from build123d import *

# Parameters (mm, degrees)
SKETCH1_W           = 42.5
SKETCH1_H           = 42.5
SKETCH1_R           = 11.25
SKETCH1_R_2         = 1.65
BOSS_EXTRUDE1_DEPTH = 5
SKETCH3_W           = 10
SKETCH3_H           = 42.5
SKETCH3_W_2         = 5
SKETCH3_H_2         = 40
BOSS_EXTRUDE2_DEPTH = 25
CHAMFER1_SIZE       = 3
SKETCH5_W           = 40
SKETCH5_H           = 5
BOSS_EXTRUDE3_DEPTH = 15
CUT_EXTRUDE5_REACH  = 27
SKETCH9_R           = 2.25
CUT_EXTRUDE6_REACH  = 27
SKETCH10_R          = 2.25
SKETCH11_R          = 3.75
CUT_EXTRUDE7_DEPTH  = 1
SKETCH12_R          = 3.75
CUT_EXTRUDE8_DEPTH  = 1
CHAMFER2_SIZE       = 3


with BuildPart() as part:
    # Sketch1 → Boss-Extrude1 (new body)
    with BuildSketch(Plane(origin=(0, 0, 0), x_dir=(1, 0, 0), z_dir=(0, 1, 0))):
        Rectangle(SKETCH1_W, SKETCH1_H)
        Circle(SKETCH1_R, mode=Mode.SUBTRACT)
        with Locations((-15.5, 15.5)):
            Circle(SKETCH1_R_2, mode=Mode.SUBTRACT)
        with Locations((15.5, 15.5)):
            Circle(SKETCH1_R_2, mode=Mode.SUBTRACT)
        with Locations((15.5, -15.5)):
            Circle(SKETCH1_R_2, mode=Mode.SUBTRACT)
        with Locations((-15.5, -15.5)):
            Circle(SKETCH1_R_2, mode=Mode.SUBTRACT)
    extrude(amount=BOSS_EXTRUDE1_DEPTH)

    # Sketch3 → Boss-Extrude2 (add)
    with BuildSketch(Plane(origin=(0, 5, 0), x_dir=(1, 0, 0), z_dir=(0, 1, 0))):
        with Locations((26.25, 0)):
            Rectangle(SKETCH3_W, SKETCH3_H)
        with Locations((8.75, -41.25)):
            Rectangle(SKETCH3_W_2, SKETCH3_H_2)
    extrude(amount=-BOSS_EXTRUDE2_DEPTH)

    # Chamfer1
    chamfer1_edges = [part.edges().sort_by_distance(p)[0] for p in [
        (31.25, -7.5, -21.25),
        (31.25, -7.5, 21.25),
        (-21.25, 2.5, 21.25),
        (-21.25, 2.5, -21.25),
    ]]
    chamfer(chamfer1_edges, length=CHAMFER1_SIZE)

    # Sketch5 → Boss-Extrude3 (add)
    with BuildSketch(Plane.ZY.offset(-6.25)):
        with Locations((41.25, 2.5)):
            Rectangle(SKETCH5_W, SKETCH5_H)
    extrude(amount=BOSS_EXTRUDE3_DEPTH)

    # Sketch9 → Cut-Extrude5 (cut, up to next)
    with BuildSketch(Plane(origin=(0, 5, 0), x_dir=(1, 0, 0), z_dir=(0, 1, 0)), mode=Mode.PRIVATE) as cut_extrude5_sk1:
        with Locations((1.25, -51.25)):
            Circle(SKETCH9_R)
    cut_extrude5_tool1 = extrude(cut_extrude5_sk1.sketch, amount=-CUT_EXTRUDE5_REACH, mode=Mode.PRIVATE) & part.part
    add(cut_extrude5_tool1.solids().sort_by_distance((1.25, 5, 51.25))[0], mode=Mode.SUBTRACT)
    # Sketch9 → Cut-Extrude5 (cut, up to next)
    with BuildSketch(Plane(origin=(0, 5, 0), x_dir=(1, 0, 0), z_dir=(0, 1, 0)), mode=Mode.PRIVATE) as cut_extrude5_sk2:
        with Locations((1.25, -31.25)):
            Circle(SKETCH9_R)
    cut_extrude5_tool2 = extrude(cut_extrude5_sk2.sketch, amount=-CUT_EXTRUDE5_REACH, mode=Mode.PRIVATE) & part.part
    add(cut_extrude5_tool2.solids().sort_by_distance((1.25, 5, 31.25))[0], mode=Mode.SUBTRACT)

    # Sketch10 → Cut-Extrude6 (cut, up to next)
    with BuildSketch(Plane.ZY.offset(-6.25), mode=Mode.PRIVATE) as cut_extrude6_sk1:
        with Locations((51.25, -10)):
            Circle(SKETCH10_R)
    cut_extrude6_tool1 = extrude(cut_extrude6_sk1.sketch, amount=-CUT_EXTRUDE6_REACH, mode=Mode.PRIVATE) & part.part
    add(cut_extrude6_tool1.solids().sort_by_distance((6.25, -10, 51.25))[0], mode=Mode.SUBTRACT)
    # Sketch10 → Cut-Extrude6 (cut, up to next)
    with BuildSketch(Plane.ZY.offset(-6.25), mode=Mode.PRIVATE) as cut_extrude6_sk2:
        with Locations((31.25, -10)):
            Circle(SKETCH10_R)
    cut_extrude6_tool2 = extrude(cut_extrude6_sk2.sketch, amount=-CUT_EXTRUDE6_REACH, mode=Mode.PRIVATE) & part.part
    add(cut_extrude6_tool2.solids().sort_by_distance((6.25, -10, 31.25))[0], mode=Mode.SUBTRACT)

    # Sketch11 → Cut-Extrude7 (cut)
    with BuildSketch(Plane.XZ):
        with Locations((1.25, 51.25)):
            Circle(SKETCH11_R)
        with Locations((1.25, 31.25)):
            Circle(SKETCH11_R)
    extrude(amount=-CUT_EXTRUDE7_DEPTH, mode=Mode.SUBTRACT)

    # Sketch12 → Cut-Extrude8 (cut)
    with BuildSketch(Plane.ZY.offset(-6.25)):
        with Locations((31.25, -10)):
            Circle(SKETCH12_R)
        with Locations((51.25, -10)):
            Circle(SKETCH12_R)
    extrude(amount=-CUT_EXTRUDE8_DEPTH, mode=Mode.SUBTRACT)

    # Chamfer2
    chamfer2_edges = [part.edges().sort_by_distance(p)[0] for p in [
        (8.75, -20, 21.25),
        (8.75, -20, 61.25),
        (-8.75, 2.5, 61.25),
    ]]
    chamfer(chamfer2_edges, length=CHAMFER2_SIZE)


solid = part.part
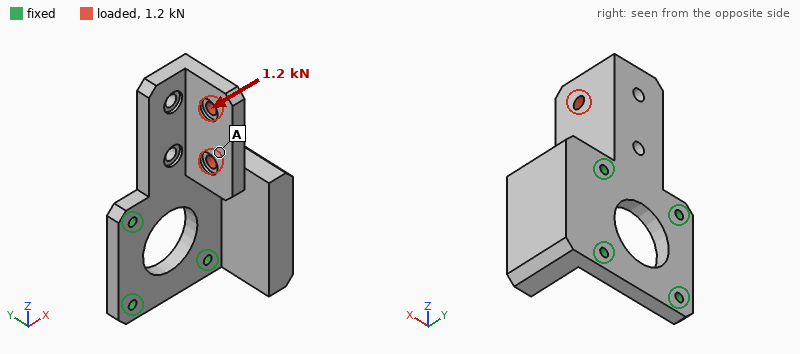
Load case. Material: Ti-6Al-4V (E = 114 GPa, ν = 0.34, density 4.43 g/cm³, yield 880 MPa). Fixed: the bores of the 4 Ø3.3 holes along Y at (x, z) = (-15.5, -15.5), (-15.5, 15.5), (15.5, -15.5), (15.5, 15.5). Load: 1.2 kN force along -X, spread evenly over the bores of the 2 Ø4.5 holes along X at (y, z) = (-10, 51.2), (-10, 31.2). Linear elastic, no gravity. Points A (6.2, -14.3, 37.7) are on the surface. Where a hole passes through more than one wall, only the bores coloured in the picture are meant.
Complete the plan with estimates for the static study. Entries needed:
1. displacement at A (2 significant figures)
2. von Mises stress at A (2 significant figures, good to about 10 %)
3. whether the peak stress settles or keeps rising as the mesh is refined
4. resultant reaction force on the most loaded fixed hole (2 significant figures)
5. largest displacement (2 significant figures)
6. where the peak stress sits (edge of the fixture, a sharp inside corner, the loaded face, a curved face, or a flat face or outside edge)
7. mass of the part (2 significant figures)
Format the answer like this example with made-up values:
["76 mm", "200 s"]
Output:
["0.15 mm", "24 MPa", "keeps rising", "1.4 kN", "0.26 mm", "a sharp inside corner", "110 g"]
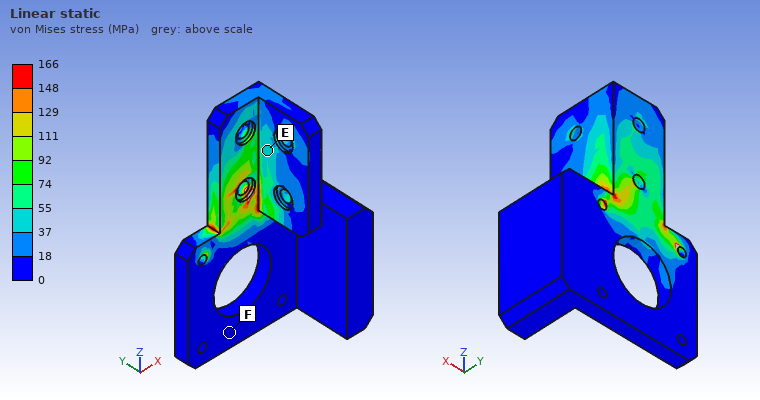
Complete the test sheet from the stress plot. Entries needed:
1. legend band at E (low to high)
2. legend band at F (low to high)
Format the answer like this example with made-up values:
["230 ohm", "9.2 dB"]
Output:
["37 to 55 MPa", "0 to 18 MPa"]
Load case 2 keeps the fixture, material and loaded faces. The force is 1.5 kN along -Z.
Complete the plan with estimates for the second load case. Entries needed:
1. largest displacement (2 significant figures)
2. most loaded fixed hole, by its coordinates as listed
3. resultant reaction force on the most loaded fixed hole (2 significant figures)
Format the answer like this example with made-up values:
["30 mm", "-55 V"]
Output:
["0.53 mm", "(15.5, 15.5)", "1.2 kN"]
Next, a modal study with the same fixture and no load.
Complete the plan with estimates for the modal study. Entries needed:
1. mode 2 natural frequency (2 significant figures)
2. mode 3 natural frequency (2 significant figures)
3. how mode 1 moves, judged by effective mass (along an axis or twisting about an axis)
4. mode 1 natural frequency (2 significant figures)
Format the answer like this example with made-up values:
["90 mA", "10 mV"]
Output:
["3300 Hz", "3600 Hz", "along Y", "1300 Hz"]
